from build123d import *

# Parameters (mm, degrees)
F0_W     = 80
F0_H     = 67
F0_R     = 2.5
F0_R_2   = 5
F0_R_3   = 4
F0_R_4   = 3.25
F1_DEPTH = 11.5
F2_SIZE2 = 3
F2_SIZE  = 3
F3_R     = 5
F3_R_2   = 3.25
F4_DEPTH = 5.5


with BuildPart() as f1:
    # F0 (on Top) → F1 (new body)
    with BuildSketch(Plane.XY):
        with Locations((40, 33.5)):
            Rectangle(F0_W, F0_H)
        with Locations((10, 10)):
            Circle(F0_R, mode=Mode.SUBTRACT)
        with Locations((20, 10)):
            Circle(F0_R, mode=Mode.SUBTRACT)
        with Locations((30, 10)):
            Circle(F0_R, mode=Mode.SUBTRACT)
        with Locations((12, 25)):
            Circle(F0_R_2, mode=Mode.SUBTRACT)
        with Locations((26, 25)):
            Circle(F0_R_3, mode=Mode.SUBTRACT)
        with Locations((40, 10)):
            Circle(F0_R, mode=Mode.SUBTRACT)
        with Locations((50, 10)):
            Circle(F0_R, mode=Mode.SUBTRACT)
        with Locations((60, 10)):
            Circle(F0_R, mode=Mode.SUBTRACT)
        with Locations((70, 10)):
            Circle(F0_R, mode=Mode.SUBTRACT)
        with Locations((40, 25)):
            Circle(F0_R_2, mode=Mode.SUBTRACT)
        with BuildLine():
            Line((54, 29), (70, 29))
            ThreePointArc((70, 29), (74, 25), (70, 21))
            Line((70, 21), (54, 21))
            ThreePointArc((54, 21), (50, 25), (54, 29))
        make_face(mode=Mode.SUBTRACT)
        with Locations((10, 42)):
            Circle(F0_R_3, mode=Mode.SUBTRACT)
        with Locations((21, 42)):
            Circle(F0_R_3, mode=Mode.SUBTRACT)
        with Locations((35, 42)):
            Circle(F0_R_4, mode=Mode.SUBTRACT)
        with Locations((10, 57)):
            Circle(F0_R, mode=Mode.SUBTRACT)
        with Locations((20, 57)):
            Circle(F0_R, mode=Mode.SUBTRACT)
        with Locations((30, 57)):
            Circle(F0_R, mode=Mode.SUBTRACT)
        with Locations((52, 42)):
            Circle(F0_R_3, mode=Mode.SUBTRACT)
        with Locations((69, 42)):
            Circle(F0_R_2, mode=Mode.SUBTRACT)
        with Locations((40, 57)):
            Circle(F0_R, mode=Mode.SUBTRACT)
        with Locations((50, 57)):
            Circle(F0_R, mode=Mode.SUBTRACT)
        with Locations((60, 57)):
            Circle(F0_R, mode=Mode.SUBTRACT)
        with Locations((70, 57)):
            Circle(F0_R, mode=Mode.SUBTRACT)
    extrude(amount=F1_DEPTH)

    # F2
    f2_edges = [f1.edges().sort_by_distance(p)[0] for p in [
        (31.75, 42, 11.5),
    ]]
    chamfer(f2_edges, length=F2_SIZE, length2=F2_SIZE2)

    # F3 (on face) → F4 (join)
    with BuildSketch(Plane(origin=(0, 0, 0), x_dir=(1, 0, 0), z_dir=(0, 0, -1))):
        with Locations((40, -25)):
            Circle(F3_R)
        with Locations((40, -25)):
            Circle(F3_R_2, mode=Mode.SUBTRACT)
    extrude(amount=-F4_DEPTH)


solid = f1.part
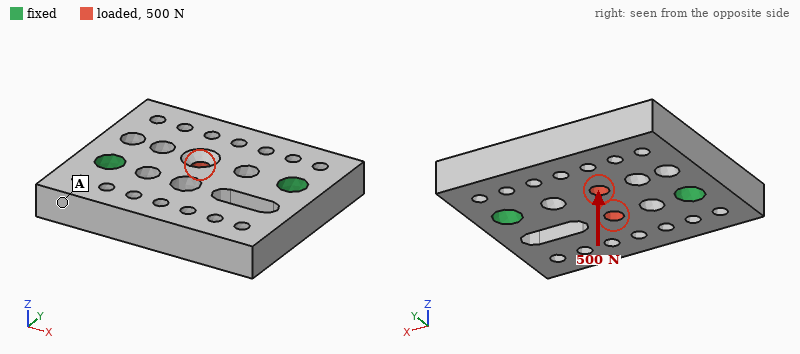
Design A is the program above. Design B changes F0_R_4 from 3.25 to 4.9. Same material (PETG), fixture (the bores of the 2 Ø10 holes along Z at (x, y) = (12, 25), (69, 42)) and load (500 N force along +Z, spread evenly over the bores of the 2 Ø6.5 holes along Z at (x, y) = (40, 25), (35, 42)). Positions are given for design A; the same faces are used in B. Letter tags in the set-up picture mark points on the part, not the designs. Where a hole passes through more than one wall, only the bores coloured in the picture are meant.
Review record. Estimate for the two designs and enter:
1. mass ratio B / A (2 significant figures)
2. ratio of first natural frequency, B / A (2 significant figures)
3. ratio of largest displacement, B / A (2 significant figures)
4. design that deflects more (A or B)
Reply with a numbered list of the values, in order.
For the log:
1. 0.99
2. 1.00
3. 1.1
4. B
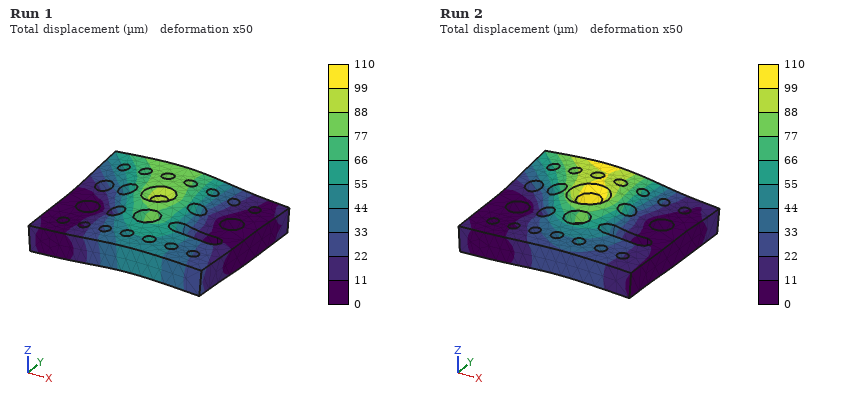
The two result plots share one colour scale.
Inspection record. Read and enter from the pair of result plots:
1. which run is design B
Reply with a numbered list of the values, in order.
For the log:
1. Run 2
